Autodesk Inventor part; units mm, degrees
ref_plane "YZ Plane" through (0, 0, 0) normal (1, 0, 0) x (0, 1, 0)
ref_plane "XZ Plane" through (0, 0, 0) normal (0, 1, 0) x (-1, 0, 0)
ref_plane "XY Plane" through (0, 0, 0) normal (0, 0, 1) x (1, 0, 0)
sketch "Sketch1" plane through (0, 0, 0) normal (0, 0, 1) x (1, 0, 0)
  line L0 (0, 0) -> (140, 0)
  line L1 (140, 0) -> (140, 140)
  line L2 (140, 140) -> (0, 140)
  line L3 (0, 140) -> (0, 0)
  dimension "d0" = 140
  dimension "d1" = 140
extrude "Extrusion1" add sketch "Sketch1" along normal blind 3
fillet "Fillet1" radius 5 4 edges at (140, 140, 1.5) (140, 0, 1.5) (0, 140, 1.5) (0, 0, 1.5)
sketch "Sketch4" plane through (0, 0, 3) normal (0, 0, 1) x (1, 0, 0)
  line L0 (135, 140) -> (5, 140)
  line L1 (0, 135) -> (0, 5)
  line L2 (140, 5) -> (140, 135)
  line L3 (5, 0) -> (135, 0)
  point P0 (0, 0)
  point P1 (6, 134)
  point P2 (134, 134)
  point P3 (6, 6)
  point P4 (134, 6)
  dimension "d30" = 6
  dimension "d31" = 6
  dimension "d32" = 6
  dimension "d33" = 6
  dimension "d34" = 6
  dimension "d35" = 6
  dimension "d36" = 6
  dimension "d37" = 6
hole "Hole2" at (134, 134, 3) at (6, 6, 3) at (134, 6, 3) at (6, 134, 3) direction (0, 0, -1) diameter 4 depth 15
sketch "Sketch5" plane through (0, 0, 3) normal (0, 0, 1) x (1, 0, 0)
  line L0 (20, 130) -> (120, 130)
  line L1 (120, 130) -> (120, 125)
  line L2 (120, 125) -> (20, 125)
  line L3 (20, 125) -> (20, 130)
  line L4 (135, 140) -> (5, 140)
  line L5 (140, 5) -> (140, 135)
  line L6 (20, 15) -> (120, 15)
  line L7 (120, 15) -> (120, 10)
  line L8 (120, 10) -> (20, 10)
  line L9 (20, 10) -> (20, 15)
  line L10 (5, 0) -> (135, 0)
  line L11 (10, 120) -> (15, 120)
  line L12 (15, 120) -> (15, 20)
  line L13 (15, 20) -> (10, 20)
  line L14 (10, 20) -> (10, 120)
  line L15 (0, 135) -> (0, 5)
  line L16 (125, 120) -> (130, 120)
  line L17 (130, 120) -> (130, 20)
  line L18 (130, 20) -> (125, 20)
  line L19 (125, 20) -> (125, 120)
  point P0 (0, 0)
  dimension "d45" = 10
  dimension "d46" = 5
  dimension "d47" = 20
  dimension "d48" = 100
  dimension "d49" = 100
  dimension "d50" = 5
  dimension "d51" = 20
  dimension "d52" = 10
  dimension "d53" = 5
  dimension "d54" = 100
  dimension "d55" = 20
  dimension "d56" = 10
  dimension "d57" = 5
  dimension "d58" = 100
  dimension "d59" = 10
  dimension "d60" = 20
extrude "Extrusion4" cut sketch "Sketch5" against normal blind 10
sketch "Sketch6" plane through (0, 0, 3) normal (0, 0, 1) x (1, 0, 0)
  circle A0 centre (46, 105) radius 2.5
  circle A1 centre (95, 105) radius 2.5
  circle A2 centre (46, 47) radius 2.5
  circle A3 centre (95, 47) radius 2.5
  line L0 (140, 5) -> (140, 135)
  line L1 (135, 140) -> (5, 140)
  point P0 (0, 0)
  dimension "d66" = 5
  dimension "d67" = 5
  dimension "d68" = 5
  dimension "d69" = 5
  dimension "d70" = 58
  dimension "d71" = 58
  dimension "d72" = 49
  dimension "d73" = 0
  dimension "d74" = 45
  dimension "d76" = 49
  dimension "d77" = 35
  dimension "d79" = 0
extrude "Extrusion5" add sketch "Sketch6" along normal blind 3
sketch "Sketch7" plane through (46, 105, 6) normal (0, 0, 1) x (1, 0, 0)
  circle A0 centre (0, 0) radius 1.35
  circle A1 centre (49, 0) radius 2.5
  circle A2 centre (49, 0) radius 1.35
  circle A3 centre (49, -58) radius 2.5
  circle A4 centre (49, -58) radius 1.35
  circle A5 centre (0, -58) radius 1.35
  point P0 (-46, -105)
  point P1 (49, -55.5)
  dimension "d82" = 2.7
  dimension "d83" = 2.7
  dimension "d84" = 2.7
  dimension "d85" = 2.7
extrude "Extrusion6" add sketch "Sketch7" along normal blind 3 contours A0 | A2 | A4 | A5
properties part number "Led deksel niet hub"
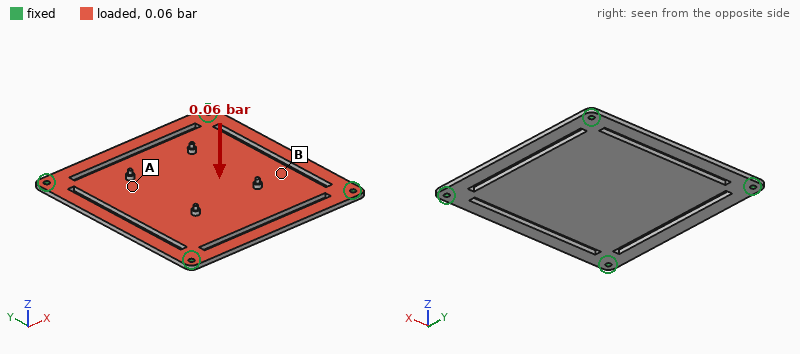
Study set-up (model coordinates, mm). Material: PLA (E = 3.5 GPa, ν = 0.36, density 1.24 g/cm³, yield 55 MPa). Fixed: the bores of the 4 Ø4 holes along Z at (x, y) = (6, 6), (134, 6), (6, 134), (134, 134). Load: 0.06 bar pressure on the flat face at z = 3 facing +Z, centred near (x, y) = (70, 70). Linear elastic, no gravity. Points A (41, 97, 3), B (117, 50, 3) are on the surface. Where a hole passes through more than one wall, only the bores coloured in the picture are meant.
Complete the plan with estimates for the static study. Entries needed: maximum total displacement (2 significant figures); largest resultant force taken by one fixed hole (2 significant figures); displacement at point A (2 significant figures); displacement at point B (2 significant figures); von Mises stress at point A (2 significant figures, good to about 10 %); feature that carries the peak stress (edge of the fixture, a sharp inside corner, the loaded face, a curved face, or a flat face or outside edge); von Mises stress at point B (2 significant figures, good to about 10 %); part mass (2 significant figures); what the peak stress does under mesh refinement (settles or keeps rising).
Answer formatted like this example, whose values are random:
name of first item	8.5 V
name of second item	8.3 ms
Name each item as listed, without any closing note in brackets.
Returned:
maximum total displacement	1.8 mm
largest resultant force taken by one fixed hole	26 N
displacement at point A	1.4 mm
displacement at point B	1.2 mm
von Mises stress at point A	3.3 MPa
feature that carries the peak stress	edge of the fixture
von Mises stress at point B	4.2 MPa
part mass	66 g
what the peak stress does under mesh refinement	keeps rising
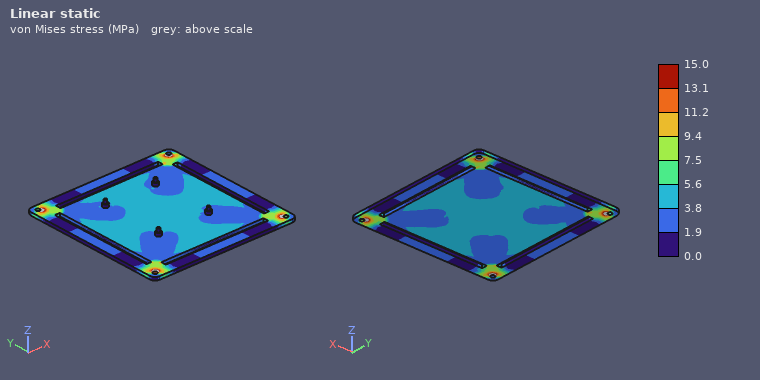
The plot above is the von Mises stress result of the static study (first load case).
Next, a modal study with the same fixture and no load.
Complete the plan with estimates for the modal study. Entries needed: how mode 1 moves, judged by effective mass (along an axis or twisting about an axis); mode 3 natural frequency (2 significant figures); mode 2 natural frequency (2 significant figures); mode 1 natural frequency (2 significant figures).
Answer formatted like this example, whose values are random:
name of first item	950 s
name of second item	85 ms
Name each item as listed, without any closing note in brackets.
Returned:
how mode 1 moves, judged by effective mass	along Z
mode 3 natural frequency	330 Hz
mode 2 natural frequency	330 Hz
mode 1 natural frequency	170 Hz
